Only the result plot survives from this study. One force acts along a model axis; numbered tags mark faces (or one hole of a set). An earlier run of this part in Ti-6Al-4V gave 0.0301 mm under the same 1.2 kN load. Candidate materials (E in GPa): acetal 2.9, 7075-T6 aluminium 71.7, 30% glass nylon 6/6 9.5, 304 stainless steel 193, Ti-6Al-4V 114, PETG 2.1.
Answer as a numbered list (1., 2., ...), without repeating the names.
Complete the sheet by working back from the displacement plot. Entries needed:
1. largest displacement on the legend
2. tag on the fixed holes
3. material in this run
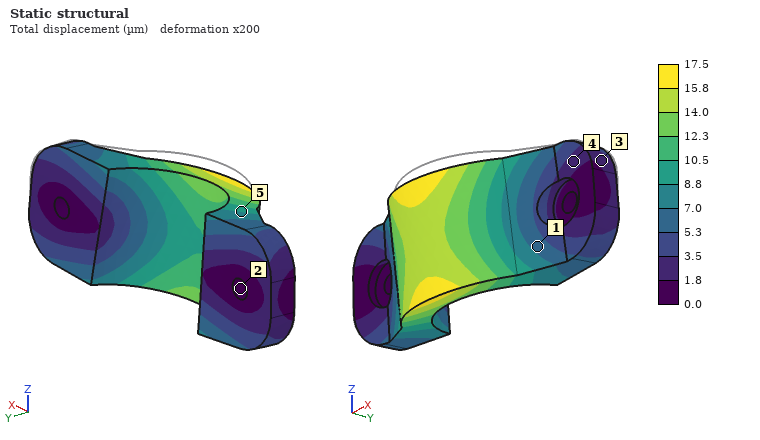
1. 17.5 µm
2. 2
3. 304 stainless steel
